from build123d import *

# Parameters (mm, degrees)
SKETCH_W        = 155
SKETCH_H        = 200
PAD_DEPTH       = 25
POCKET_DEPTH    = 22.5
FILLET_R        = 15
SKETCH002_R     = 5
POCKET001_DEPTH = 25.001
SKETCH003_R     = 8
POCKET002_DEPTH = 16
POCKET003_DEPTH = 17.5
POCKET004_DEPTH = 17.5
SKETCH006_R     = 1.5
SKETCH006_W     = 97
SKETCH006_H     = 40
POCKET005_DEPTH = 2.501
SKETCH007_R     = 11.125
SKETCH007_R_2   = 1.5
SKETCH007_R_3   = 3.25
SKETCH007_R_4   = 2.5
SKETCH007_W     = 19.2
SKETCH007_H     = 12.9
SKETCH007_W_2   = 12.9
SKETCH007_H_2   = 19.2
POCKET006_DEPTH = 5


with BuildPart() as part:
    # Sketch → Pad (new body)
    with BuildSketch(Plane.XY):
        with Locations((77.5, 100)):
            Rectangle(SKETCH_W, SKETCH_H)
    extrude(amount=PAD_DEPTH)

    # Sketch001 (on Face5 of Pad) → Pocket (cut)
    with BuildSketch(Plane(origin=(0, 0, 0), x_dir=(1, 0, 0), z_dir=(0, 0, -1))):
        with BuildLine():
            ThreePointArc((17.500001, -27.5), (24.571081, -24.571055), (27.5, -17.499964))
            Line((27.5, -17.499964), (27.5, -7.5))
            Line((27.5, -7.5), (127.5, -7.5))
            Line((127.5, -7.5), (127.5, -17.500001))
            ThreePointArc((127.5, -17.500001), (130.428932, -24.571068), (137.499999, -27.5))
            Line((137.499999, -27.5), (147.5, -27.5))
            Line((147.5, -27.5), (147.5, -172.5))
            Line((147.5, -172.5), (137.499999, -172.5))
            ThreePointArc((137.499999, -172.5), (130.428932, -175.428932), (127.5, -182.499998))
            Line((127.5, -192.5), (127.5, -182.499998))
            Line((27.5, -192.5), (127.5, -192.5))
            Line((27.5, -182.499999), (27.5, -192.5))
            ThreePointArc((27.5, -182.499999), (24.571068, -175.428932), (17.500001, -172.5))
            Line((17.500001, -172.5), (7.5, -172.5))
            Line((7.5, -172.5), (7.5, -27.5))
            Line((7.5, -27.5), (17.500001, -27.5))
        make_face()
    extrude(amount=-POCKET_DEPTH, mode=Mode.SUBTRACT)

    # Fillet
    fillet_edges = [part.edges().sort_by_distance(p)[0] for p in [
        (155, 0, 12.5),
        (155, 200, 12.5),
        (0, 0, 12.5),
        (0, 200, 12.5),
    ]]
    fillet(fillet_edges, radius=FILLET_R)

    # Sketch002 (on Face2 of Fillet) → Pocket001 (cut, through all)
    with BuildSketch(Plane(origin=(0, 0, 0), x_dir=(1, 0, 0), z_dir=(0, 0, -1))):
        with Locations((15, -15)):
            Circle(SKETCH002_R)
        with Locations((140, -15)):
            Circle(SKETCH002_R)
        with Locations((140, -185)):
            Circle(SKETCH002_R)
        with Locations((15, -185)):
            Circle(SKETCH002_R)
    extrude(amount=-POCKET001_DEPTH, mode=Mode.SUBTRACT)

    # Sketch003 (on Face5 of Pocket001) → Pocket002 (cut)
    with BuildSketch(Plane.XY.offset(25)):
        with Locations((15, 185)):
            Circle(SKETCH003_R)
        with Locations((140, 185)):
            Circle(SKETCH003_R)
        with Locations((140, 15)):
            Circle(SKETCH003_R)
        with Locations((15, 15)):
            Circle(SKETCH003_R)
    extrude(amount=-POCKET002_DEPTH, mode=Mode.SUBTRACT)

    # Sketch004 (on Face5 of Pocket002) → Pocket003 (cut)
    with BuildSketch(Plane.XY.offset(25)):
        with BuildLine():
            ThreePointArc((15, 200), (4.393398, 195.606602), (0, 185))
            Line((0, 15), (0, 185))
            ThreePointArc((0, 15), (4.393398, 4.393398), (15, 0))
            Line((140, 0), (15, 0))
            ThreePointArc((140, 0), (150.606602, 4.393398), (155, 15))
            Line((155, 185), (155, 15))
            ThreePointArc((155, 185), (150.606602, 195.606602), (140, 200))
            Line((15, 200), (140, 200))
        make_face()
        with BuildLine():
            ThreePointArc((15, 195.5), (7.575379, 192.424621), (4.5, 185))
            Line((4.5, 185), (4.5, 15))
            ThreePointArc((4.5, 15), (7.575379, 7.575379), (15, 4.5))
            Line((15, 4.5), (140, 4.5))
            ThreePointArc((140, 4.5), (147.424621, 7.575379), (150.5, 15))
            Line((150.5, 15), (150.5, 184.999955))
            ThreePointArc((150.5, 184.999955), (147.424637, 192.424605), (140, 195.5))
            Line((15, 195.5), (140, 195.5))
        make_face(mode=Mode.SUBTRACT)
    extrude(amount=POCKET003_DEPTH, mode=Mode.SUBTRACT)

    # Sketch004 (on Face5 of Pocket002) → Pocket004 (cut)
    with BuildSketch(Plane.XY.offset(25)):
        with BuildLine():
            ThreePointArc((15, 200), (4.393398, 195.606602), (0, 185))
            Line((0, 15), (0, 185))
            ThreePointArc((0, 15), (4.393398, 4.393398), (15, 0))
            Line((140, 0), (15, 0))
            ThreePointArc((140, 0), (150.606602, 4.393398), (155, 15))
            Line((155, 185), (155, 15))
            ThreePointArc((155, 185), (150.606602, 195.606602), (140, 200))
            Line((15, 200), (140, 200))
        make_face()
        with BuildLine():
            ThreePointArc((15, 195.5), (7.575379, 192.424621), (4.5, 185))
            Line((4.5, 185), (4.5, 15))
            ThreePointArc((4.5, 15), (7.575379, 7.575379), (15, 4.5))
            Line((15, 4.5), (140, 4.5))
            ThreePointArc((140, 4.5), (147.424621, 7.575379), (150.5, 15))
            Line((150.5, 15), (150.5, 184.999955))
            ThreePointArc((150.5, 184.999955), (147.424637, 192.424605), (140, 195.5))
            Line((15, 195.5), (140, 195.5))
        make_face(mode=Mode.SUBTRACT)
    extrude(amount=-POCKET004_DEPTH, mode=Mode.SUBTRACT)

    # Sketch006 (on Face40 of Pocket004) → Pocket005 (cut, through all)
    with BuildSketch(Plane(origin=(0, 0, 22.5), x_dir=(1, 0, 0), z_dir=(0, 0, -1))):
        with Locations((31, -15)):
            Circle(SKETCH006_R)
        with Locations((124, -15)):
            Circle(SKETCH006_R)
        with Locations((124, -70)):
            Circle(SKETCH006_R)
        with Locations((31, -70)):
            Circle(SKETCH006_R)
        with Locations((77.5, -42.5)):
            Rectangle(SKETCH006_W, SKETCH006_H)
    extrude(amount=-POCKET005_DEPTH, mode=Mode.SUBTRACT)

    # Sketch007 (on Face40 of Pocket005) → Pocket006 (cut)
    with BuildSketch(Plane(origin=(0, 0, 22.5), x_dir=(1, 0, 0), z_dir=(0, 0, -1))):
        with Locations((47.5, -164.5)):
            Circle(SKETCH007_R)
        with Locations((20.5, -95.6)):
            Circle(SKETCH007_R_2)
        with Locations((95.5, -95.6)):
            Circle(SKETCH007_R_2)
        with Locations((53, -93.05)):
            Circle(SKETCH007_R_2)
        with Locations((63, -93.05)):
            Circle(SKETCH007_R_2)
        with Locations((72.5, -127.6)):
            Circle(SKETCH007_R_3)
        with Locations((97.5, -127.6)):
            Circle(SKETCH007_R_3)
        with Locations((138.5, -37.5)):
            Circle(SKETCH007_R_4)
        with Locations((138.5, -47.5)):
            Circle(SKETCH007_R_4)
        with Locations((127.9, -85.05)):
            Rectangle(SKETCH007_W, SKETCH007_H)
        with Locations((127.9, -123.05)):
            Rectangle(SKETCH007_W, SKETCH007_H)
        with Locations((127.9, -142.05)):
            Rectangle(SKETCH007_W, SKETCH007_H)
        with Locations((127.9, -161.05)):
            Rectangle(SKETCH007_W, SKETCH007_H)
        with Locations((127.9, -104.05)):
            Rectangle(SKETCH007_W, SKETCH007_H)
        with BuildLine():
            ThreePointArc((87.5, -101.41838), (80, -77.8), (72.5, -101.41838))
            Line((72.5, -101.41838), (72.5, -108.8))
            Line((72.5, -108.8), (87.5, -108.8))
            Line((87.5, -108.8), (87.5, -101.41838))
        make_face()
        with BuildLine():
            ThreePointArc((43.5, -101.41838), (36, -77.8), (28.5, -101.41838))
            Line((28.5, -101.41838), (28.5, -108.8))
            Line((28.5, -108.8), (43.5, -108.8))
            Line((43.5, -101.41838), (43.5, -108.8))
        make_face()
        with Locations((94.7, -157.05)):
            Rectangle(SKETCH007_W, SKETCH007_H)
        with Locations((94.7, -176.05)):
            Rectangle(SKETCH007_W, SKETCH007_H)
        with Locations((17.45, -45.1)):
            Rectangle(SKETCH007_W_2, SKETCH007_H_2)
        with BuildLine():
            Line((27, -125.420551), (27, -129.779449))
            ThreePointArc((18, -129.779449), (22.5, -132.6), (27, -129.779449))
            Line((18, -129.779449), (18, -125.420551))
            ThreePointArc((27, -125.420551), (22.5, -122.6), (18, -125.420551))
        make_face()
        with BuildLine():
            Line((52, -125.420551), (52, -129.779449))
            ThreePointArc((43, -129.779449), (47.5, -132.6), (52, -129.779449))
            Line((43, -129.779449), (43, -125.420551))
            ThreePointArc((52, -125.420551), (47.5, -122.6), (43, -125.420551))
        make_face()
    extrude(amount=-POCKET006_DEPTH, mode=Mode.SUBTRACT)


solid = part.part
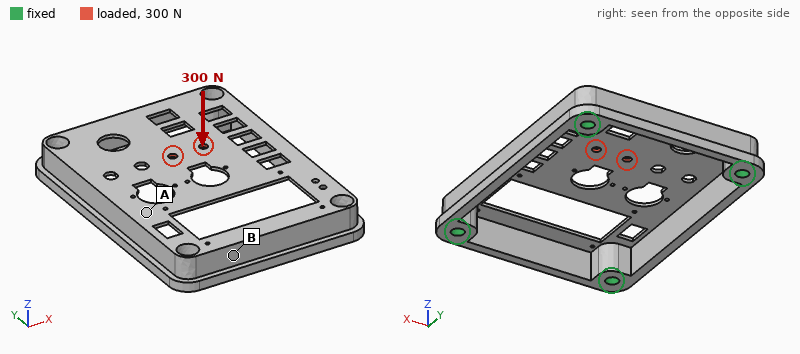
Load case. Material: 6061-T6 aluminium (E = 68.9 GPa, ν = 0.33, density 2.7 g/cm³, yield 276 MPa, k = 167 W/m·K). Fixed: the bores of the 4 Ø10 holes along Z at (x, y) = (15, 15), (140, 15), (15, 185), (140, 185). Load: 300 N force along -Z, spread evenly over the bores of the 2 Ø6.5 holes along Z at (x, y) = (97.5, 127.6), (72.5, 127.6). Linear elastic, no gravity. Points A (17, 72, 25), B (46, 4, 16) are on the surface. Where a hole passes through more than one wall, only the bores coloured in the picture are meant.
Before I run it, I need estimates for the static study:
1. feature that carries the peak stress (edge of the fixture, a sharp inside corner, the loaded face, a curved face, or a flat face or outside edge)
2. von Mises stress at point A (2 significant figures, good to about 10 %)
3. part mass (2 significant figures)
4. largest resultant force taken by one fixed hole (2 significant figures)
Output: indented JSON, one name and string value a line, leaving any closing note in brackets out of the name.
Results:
{
  "feature that carries the peak stress": "the loaded face",
  "von Mises stress at point A": "15 MPa",
  "part mass": "360 g",
  "largest resultant force taken by one fixed hole": "150 N"
}
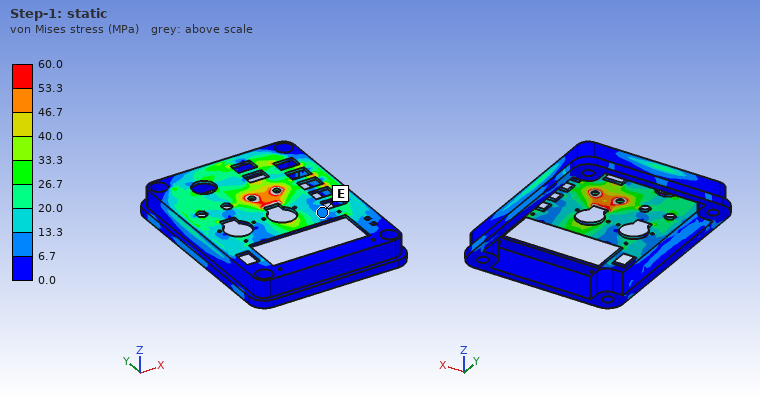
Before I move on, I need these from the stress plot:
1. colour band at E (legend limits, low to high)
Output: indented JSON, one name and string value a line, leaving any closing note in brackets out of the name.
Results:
{
  "colour band at E": "6.7 to 13.3 MPa"
}
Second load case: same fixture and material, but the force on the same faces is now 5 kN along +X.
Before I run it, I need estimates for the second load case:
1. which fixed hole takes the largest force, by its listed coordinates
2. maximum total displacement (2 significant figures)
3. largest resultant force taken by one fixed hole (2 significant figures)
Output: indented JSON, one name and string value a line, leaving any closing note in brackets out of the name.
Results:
{
  "which fixed hole takes the largest force, by its listed coordinates": "(15, 185)",
  "maximum total displacement": "0.11 mm",
  "largest resultant force taken by one fixed hole": "2.5 kN"
}
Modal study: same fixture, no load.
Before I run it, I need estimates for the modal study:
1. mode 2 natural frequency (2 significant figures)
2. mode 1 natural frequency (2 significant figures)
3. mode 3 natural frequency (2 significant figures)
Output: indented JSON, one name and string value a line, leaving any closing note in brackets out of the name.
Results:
{
  "mode 2 natural frequency": "1200 Hz",
  "mode 1 natural frequency": "650 Hz",
  "mode 3 natural frequency": "1600 Hz"
}
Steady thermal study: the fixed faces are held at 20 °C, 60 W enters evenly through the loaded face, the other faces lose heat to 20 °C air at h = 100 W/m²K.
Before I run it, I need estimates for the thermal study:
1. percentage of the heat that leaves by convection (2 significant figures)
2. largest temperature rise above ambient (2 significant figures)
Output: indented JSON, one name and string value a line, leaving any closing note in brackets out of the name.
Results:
{
  "percentage of the heat that leaves by convection": "80 %",
  "largest temperature rise above ambient": "53 K"
}
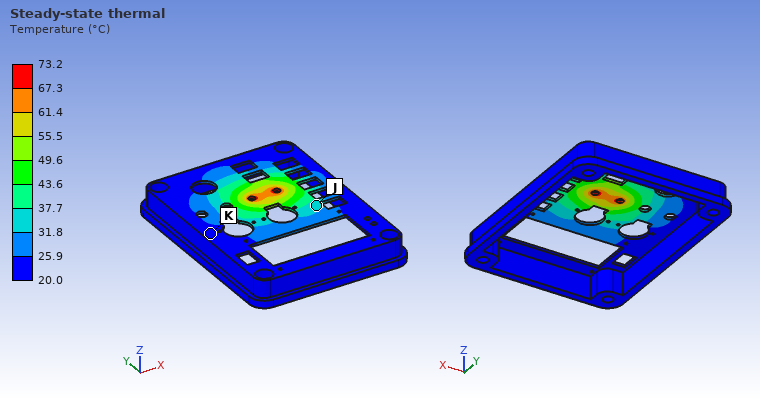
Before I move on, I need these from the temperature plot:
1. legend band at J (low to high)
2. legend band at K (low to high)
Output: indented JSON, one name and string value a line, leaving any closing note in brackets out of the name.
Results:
{
  "legend band at J": "31.8 to 37.7 °C",
  "legend band at K": "20.0 to 25.9 °C"
}
